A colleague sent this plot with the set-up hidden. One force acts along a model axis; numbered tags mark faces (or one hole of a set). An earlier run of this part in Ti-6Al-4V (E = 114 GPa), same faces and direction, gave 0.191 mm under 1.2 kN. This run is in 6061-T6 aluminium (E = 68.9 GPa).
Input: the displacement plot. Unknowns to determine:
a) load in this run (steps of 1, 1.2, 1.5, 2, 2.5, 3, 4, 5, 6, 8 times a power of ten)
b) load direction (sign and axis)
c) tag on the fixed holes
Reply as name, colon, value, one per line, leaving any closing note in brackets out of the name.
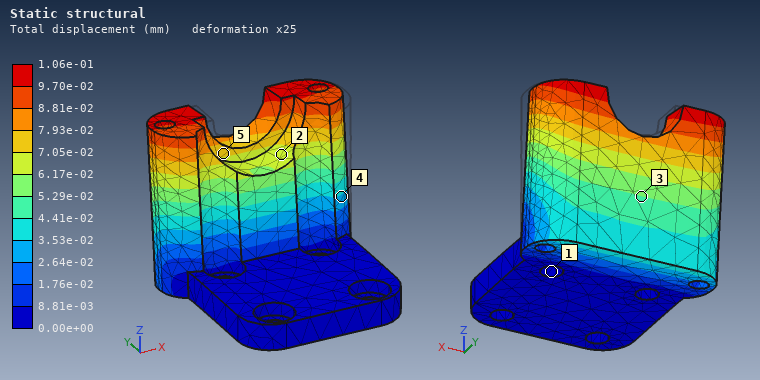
load in this run: 400 N
load direction: +Y
tag on the fixed holes: 1
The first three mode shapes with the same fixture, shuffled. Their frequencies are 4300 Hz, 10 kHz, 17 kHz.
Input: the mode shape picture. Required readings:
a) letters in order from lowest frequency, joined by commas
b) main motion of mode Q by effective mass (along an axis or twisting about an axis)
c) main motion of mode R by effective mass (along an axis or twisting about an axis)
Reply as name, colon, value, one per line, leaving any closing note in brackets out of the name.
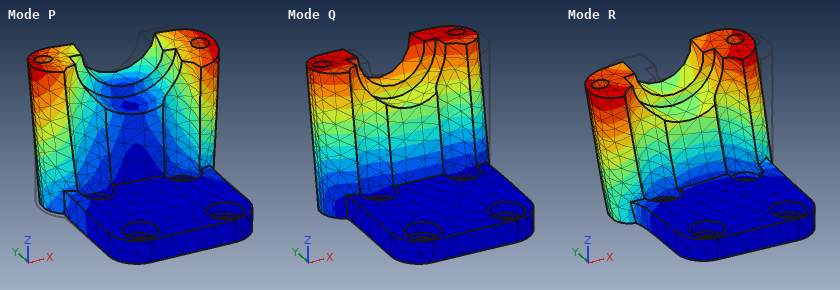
letters in order from lowest frequency, joined by commas: Q, R, P
main motion of mode Q by effective mass: along Y
main motion of mode R by effective mass: along X
